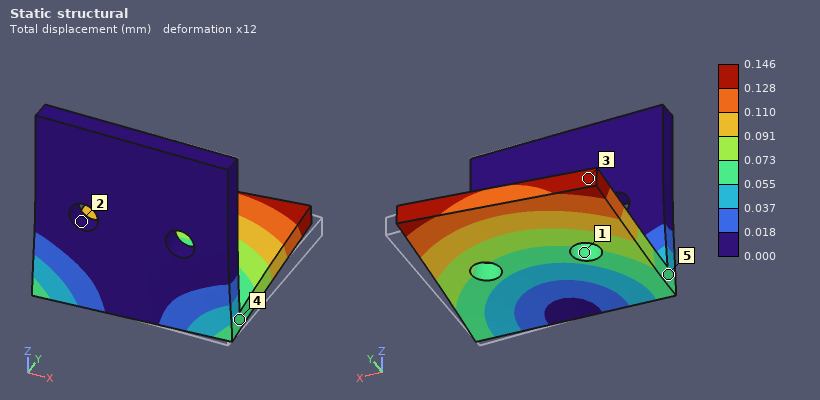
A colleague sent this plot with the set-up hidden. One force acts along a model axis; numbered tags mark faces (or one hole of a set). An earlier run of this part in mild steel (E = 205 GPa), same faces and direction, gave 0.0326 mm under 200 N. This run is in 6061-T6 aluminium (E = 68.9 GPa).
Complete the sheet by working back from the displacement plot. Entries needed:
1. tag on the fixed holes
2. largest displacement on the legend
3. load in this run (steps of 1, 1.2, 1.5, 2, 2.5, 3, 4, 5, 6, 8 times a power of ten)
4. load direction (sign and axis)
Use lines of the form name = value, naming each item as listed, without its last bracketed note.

tag on the fixed holes = 2
largest displacement on the legend = 0.146 mm
load in this run = 300 N
load direction = -X
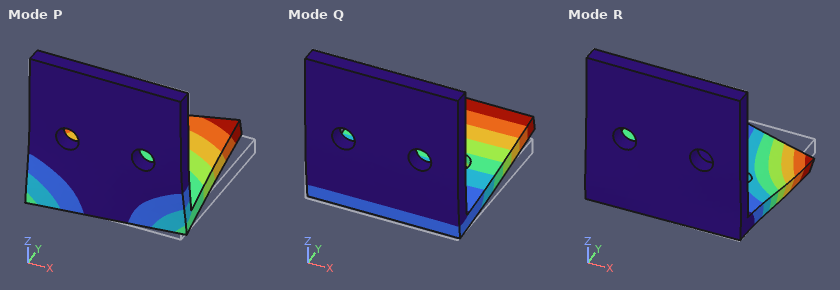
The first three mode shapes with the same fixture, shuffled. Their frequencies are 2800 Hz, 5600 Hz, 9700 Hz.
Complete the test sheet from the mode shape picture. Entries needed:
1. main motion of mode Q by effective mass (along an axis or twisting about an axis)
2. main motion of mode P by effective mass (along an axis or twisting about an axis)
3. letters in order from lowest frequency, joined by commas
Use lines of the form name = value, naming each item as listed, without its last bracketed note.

main motion of mode Q by effective mass = along Z
main motion of mode P by effective mass = along X
letters in order from lowest frequency, joined by commas = Q, P, R
